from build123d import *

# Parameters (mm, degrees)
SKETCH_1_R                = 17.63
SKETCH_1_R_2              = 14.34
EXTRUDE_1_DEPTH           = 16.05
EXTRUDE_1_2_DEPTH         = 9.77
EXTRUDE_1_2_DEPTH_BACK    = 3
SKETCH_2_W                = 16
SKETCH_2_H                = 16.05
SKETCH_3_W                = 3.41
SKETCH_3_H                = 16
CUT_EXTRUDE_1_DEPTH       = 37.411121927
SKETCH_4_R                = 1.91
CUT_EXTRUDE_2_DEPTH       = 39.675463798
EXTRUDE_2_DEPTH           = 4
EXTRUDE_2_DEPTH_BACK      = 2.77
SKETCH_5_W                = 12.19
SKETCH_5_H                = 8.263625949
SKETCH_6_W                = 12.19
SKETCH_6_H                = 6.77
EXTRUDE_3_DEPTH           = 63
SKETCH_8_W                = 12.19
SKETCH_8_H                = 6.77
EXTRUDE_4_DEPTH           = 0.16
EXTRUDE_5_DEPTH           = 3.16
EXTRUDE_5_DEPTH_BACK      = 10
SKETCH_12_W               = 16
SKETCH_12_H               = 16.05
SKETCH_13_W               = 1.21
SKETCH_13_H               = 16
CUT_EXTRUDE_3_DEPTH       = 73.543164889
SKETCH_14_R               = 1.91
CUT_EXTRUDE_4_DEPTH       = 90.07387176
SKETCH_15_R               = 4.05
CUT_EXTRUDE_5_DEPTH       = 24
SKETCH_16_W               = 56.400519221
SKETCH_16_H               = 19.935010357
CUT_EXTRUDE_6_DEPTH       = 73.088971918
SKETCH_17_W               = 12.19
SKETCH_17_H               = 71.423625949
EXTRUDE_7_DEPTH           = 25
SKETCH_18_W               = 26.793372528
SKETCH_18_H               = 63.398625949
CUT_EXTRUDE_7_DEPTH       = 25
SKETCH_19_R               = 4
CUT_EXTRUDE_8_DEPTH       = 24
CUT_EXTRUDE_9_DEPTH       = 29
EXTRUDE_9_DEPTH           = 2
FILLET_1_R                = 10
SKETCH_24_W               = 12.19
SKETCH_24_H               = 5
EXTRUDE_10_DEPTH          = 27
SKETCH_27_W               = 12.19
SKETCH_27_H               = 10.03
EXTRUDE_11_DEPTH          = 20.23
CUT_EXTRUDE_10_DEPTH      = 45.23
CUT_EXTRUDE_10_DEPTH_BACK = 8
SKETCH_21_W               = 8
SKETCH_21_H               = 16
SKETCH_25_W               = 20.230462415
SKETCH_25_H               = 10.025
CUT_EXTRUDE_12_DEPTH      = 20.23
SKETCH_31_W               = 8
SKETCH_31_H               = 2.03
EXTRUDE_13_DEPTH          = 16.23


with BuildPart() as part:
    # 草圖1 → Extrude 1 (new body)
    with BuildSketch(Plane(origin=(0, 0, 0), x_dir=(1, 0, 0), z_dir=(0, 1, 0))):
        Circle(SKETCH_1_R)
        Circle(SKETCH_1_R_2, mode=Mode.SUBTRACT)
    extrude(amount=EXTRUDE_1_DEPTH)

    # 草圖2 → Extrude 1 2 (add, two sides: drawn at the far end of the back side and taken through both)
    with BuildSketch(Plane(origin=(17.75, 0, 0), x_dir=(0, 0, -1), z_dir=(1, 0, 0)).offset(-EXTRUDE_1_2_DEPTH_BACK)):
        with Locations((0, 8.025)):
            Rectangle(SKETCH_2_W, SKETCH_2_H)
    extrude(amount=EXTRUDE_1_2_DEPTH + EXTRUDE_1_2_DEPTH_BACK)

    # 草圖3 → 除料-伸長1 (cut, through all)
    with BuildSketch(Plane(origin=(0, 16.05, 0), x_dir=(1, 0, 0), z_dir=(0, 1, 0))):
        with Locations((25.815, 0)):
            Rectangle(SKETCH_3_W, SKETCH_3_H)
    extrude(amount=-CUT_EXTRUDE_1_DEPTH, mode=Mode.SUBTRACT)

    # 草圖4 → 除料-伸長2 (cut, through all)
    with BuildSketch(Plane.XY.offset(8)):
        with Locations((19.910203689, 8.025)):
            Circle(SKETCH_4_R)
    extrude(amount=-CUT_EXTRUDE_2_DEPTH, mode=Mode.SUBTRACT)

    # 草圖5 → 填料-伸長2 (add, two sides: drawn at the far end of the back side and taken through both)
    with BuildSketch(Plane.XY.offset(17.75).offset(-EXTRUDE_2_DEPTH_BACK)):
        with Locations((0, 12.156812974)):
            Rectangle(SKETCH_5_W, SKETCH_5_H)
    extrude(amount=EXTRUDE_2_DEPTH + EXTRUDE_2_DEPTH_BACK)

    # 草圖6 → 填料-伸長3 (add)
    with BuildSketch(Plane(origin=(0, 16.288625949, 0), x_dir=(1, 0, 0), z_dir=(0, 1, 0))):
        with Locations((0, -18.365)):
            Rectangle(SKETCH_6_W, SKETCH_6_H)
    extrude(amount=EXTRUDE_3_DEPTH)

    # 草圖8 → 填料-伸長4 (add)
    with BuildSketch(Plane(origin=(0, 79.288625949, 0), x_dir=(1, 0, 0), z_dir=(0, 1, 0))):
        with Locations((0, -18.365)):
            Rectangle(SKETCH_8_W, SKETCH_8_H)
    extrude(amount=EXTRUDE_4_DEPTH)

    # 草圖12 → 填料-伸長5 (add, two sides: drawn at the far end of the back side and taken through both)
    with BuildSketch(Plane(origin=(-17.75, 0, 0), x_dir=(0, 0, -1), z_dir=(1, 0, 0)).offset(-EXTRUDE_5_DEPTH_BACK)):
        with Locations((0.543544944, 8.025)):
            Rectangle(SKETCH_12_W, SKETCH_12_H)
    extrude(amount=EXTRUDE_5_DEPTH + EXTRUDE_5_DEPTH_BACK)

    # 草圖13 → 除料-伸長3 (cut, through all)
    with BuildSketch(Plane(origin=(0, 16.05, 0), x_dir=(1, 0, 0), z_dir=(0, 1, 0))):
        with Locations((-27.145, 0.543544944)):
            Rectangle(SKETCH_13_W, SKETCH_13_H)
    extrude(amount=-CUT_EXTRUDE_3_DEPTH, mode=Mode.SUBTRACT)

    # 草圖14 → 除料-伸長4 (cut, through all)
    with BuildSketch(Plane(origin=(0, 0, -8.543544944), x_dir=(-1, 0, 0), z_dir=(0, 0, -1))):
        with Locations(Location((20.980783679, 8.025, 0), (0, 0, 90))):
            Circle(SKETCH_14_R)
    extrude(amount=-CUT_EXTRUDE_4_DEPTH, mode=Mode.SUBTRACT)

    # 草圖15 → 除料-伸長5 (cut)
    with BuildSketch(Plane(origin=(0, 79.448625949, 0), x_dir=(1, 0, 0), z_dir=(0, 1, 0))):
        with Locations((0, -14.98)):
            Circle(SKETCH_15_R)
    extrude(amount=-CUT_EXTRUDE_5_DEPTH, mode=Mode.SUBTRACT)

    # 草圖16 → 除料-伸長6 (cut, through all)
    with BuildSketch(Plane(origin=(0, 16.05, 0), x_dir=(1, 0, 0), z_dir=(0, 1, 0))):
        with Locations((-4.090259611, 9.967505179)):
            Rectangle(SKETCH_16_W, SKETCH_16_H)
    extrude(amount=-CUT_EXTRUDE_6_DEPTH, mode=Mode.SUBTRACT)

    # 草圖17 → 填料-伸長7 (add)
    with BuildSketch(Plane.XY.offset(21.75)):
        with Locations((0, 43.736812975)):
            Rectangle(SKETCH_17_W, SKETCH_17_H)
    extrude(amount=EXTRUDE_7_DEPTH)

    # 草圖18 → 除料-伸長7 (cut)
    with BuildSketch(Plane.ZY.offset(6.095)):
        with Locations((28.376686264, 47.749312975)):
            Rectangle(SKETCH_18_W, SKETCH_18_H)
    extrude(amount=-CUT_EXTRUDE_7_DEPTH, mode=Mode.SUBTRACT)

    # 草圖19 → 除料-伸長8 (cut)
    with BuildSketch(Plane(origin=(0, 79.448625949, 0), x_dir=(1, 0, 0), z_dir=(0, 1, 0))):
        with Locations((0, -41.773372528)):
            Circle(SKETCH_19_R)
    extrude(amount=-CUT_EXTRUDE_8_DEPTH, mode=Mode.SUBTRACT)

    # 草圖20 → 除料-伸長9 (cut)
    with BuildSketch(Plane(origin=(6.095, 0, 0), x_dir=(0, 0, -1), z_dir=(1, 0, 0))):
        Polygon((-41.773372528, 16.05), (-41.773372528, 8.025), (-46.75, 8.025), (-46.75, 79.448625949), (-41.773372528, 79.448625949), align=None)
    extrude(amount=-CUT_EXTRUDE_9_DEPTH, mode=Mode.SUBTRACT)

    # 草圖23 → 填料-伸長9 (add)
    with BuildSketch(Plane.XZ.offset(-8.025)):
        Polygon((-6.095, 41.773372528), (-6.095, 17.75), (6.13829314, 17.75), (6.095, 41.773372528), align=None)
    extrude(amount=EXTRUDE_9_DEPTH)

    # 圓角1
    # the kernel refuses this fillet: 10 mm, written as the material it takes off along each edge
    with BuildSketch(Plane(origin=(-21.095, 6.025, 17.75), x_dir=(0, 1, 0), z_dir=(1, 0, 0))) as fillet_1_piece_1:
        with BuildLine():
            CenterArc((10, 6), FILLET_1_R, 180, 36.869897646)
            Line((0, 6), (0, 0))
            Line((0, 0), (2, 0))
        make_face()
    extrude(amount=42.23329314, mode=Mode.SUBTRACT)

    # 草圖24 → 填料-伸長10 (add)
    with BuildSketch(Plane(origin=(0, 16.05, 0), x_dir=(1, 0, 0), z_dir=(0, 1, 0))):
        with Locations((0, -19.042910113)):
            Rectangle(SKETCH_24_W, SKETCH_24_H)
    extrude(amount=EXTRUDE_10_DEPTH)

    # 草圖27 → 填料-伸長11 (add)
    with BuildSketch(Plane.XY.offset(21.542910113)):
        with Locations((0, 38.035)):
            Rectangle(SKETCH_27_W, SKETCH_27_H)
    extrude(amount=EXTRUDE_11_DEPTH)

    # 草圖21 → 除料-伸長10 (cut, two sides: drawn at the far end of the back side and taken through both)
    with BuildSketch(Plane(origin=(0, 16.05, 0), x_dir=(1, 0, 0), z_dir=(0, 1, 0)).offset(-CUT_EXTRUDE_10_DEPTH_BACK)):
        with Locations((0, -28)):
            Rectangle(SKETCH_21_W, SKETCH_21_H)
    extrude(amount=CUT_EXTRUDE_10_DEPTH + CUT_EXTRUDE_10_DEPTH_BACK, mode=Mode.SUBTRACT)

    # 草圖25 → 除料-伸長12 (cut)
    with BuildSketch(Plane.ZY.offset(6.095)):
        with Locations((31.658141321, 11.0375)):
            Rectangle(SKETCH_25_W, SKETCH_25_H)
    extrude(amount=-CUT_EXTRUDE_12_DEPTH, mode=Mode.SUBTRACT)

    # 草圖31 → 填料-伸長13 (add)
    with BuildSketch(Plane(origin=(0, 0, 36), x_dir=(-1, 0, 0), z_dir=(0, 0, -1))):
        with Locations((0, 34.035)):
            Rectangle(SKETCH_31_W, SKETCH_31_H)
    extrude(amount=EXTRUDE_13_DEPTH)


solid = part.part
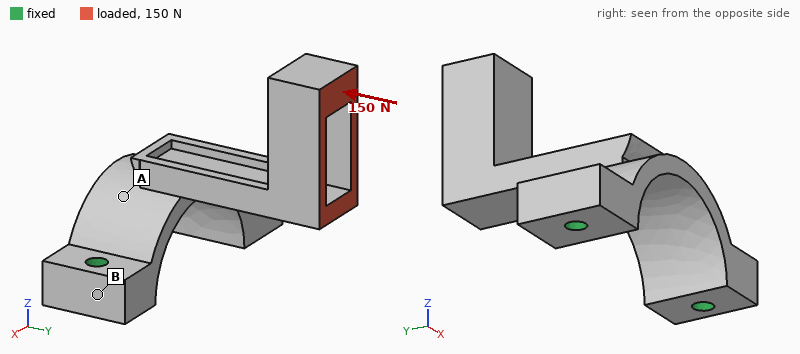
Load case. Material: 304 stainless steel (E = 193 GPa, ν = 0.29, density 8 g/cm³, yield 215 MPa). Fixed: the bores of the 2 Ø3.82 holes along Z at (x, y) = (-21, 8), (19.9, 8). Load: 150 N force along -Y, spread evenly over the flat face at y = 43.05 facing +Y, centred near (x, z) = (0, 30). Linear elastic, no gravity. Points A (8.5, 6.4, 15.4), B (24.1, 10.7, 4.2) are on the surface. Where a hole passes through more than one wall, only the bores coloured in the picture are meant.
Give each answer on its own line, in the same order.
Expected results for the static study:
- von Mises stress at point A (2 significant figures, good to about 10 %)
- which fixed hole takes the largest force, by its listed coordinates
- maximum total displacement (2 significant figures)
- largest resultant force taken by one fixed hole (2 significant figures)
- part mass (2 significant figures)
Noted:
15 MPa
(19.9, 8)
99 µm
82 N
62 g
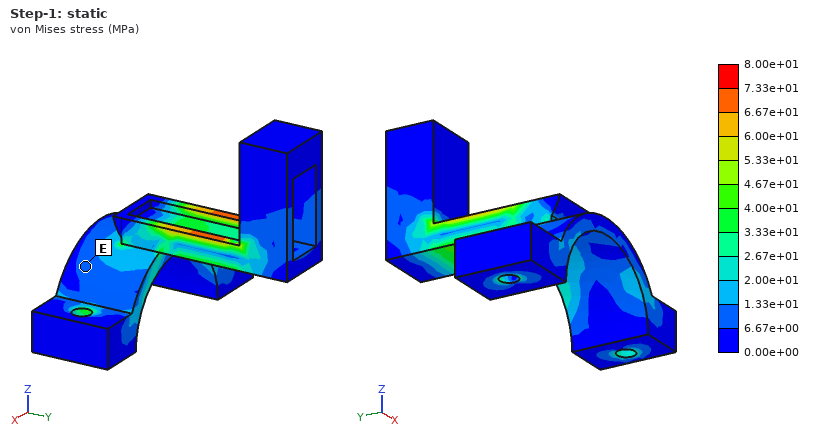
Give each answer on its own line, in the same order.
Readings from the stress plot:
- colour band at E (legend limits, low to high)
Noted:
6.67e+00 to 1.33e+01 MPa
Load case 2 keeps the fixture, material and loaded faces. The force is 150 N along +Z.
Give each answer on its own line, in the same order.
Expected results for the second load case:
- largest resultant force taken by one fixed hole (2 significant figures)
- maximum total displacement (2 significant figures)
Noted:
110 N
0.17 mm
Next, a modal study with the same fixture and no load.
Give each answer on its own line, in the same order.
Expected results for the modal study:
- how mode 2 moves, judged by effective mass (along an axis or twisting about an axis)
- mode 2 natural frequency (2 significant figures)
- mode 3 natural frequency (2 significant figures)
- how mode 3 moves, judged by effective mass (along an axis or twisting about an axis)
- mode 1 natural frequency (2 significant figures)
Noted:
along X
2100 Hz
5600 Hz
along Z
1400 Hz
